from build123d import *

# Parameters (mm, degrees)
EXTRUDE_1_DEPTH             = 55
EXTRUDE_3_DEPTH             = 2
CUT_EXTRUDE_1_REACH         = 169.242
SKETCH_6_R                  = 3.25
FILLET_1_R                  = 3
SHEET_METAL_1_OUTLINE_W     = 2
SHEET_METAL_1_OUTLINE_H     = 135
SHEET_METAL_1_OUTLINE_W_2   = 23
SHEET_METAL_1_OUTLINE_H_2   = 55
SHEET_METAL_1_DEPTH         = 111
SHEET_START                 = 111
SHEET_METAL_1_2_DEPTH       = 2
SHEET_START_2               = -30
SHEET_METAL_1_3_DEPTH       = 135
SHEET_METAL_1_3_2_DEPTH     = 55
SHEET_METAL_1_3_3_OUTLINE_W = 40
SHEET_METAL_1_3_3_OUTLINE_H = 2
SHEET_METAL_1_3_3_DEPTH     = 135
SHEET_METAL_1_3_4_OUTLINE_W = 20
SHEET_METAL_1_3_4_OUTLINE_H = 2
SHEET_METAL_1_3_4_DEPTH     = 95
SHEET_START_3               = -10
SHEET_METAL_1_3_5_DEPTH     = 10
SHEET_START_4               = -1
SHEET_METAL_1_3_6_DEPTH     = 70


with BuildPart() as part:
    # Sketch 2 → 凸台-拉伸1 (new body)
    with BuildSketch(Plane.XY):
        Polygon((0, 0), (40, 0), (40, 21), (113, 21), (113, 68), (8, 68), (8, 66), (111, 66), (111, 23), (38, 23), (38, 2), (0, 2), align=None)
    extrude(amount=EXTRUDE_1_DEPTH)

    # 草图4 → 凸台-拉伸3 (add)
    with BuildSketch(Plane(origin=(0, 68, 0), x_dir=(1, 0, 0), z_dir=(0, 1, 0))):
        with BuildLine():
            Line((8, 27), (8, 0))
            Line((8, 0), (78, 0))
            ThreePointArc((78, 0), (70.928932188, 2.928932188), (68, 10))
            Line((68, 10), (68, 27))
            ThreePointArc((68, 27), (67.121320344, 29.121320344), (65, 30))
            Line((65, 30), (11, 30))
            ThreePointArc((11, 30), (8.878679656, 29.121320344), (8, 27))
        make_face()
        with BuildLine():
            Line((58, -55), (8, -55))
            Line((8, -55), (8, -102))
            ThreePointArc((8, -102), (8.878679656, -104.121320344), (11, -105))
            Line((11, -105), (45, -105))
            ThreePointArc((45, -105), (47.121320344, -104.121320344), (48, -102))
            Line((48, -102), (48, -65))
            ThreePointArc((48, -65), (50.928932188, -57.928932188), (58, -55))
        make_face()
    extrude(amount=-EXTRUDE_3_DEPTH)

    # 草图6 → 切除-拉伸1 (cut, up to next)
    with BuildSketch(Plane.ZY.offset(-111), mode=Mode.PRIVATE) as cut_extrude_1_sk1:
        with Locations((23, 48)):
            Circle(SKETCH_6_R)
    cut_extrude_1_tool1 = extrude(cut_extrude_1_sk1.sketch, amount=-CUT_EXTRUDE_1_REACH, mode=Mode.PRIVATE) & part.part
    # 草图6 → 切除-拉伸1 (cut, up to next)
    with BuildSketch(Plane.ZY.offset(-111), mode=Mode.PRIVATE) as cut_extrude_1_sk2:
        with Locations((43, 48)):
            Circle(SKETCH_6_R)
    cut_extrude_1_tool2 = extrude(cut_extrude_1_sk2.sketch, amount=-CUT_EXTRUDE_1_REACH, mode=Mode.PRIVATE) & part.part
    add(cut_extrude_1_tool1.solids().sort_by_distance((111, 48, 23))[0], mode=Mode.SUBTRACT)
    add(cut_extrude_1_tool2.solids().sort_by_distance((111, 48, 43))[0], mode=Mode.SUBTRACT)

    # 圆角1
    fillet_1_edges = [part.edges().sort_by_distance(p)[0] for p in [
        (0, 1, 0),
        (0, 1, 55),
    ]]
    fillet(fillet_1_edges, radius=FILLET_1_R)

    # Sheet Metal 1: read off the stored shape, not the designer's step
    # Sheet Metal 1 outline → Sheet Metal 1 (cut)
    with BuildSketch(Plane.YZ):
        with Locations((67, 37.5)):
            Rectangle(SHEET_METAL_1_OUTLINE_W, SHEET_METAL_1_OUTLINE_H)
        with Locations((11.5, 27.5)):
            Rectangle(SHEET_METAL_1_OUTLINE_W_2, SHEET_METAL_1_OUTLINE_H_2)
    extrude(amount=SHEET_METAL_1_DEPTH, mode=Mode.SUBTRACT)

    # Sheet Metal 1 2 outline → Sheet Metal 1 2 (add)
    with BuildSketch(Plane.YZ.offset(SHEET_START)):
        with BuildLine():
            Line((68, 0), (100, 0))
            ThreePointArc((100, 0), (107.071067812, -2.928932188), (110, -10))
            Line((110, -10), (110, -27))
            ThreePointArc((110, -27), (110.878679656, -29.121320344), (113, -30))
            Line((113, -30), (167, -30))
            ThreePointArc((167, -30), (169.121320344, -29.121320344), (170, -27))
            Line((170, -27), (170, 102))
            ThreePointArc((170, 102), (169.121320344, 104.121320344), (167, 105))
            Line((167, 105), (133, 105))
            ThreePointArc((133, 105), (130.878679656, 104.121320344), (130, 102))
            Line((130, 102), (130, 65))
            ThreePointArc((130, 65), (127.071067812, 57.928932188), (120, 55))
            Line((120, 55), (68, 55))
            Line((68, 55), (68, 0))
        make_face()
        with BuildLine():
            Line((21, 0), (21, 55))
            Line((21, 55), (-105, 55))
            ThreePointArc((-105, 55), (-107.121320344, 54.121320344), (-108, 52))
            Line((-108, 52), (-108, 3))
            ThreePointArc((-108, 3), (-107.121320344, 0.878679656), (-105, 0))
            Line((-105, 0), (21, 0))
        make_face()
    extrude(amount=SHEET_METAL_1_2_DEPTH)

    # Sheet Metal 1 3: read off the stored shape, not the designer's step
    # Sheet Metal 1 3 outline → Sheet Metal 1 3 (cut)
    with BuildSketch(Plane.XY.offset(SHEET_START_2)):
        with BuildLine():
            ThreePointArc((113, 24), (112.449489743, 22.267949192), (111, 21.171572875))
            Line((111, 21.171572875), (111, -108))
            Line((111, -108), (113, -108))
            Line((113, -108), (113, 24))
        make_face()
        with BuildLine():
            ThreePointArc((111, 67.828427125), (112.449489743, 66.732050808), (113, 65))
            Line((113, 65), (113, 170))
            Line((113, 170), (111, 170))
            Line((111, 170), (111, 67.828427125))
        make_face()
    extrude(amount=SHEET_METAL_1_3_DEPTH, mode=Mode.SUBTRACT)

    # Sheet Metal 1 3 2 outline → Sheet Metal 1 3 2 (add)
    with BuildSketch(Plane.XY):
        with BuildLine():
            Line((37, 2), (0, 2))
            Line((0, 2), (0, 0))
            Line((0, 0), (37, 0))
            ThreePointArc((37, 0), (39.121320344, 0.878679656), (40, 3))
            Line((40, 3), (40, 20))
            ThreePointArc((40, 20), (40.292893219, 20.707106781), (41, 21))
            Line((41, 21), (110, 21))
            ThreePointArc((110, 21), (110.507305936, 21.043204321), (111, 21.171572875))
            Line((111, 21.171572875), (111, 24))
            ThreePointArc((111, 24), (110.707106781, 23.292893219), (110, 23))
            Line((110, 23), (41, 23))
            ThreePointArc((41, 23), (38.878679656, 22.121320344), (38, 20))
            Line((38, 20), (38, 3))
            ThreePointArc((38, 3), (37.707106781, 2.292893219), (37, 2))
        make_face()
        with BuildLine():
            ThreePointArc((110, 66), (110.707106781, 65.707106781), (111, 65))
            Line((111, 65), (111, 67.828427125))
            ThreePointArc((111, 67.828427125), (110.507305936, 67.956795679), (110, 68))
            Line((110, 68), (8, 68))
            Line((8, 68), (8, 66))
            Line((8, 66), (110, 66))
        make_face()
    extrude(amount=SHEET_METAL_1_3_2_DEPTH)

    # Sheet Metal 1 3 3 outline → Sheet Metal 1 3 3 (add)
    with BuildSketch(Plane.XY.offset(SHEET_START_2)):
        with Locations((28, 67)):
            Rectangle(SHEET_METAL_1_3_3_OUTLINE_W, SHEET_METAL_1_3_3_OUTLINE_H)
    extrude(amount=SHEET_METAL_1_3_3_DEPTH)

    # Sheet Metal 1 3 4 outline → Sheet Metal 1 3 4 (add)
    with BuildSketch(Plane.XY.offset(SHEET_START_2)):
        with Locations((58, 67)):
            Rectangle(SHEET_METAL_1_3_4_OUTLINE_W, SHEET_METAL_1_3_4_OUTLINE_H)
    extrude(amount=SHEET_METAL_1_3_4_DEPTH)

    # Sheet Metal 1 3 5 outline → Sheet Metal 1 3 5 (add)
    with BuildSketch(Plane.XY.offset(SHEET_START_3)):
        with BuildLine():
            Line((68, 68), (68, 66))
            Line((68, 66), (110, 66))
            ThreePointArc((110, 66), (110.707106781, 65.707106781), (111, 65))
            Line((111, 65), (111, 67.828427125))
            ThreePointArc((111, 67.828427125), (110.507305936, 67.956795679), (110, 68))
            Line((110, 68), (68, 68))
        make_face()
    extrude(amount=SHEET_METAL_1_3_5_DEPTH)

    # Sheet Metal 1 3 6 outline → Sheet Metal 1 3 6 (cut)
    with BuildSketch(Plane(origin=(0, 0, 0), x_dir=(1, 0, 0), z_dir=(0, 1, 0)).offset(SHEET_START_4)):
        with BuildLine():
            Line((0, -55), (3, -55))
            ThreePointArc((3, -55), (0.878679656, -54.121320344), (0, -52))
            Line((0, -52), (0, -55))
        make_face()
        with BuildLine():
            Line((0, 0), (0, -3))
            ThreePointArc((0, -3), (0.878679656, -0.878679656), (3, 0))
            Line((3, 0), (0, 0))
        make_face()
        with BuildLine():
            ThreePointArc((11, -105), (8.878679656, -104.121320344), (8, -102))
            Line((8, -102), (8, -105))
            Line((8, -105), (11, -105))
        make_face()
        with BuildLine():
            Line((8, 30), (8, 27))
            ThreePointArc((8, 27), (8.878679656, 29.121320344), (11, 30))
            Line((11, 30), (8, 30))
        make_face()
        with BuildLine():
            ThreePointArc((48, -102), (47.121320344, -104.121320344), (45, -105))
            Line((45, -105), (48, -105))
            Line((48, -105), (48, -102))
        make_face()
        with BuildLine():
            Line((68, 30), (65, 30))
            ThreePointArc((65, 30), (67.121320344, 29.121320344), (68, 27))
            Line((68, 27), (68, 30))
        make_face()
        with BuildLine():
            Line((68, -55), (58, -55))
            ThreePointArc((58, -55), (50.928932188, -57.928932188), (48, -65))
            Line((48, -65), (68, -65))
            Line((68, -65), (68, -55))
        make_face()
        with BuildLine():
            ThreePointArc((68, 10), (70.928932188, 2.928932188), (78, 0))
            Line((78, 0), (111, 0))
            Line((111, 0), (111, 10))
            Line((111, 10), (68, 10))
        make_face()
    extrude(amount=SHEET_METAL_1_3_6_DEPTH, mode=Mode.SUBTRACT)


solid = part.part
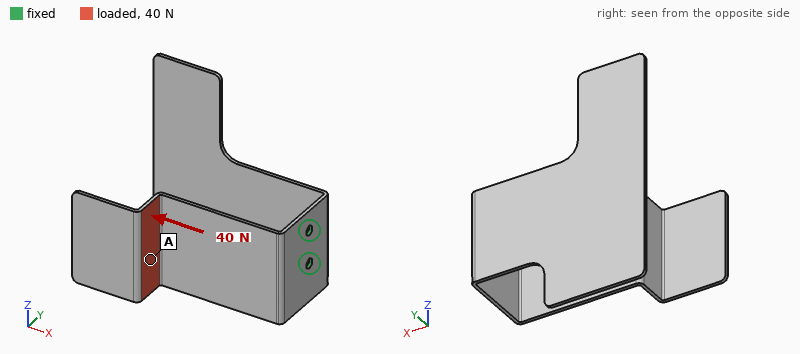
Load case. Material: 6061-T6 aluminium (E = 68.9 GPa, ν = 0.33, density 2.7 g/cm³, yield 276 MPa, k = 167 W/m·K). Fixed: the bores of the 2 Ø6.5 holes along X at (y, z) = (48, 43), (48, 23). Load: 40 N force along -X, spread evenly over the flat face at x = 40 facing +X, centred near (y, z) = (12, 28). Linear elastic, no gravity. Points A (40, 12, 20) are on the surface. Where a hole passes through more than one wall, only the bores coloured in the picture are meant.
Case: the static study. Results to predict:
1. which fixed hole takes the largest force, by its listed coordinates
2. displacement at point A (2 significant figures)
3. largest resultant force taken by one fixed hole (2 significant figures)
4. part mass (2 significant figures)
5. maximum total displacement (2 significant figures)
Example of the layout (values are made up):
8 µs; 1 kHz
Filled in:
(48, 23); 1.0 mm; 24 N; 100 g; 1.9 mm
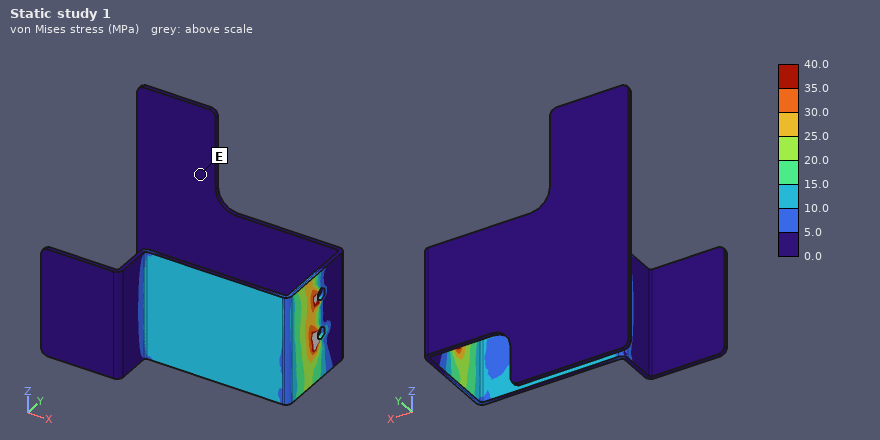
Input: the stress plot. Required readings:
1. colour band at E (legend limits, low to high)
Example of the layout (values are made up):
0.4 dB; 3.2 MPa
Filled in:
0.0 to 5.0 MPa
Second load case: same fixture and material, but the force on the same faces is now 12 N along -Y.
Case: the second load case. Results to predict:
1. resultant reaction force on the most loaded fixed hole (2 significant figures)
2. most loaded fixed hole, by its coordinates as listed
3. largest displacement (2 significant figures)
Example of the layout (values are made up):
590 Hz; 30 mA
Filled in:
9.4 N; (48, 23); 1.9 mm
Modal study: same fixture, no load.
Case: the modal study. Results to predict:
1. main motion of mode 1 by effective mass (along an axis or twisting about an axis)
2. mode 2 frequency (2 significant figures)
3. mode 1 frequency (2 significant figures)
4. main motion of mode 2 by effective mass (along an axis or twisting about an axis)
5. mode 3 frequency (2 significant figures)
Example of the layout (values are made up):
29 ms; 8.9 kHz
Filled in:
along Y; 86 Hz; 80 Hz; along Y; 170 Hz
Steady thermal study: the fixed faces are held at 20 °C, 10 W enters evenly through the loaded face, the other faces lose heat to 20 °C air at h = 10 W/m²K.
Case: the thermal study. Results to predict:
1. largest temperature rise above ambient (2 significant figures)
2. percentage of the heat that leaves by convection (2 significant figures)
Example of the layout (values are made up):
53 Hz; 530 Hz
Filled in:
39 K; 42 %
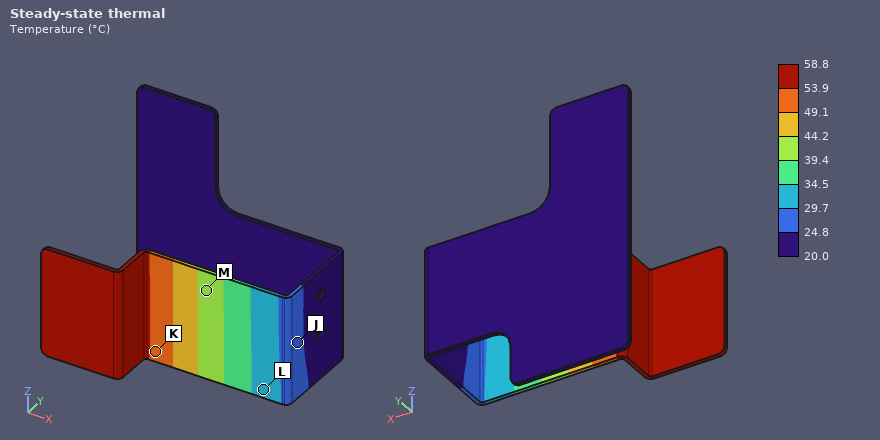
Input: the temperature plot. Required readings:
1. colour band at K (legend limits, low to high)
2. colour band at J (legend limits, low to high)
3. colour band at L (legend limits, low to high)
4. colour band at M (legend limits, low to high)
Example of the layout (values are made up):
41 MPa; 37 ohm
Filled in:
49.1 to 53.9 °C; 24.8 to 29.7 °C; 29.7 to 34.5 °C; 39.4 to 44.2 °C
